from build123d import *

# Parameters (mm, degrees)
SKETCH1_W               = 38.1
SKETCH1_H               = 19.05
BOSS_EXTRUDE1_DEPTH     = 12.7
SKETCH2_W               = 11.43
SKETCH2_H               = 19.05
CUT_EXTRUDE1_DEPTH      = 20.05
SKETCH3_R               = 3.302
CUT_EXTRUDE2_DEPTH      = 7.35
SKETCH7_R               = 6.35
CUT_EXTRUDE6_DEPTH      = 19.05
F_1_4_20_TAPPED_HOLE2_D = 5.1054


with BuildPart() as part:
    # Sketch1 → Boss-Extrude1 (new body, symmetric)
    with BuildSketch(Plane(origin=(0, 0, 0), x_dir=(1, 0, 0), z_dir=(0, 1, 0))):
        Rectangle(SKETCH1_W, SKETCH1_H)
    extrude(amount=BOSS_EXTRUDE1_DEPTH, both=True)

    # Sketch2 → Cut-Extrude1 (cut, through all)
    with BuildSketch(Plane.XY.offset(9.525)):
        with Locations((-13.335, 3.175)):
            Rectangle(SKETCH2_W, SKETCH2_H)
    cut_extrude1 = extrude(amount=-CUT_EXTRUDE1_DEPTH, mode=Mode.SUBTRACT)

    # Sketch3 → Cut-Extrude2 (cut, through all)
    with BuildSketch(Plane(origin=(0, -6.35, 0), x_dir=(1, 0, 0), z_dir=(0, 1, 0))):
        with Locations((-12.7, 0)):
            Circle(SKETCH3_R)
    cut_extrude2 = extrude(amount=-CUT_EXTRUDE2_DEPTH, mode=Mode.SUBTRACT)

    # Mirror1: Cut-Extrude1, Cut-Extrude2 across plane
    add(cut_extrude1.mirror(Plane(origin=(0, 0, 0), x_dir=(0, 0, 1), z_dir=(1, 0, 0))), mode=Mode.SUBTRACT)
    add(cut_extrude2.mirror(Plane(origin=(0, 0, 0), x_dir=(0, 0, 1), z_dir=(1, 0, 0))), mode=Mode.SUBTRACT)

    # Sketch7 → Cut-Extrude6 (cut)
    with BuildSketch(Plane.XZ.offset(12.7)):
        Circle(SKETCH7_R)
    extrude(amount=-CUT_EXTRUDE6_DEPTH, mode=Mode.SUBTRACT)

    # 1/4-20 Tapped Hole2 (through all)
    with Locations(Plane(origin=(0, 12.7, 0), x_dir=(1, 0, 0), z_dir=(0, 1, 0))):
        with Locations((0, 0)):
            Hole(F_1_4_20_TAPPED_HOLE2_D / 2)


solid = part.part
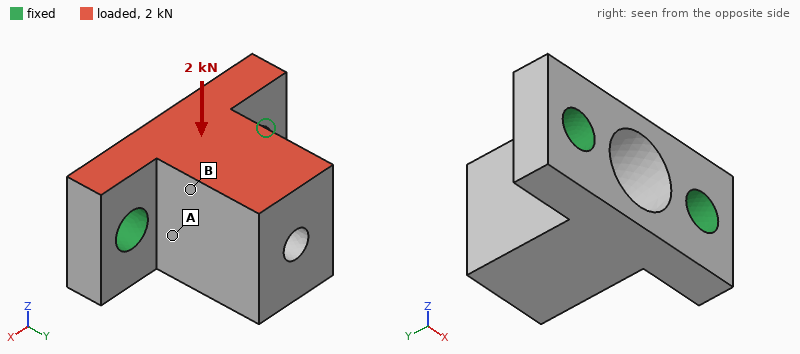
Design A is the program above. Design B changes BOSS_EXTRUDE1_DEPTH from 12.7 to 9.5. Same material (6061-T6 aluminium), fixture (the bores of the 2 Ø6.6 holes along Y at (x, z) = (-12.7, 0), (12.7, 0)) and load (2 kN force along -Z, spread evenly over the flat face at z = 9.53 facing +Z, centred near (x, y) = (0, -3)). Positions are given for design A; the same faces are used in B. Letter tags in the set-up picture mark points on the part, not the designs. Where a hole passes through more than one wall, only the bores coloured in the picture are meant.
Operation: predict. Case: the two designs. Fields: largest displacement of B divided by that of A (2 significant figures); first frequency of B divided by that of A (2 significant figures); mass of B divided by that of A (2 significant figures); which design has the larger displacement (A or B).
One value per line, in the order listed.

2.4
0.79
0.64
B
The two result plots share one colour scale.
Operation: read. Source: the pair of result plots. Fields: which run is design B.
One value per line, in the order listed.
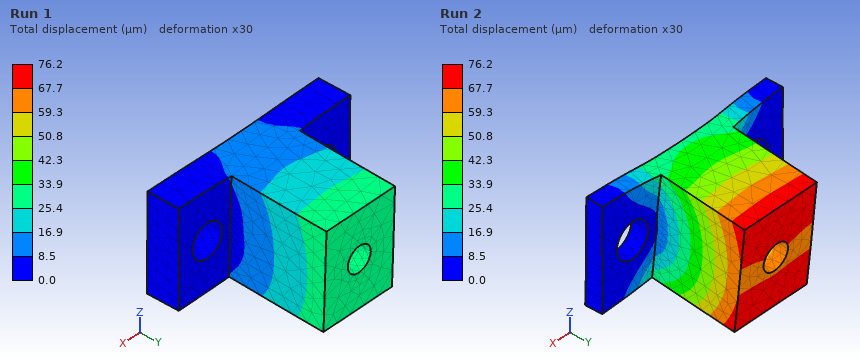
Run 2
